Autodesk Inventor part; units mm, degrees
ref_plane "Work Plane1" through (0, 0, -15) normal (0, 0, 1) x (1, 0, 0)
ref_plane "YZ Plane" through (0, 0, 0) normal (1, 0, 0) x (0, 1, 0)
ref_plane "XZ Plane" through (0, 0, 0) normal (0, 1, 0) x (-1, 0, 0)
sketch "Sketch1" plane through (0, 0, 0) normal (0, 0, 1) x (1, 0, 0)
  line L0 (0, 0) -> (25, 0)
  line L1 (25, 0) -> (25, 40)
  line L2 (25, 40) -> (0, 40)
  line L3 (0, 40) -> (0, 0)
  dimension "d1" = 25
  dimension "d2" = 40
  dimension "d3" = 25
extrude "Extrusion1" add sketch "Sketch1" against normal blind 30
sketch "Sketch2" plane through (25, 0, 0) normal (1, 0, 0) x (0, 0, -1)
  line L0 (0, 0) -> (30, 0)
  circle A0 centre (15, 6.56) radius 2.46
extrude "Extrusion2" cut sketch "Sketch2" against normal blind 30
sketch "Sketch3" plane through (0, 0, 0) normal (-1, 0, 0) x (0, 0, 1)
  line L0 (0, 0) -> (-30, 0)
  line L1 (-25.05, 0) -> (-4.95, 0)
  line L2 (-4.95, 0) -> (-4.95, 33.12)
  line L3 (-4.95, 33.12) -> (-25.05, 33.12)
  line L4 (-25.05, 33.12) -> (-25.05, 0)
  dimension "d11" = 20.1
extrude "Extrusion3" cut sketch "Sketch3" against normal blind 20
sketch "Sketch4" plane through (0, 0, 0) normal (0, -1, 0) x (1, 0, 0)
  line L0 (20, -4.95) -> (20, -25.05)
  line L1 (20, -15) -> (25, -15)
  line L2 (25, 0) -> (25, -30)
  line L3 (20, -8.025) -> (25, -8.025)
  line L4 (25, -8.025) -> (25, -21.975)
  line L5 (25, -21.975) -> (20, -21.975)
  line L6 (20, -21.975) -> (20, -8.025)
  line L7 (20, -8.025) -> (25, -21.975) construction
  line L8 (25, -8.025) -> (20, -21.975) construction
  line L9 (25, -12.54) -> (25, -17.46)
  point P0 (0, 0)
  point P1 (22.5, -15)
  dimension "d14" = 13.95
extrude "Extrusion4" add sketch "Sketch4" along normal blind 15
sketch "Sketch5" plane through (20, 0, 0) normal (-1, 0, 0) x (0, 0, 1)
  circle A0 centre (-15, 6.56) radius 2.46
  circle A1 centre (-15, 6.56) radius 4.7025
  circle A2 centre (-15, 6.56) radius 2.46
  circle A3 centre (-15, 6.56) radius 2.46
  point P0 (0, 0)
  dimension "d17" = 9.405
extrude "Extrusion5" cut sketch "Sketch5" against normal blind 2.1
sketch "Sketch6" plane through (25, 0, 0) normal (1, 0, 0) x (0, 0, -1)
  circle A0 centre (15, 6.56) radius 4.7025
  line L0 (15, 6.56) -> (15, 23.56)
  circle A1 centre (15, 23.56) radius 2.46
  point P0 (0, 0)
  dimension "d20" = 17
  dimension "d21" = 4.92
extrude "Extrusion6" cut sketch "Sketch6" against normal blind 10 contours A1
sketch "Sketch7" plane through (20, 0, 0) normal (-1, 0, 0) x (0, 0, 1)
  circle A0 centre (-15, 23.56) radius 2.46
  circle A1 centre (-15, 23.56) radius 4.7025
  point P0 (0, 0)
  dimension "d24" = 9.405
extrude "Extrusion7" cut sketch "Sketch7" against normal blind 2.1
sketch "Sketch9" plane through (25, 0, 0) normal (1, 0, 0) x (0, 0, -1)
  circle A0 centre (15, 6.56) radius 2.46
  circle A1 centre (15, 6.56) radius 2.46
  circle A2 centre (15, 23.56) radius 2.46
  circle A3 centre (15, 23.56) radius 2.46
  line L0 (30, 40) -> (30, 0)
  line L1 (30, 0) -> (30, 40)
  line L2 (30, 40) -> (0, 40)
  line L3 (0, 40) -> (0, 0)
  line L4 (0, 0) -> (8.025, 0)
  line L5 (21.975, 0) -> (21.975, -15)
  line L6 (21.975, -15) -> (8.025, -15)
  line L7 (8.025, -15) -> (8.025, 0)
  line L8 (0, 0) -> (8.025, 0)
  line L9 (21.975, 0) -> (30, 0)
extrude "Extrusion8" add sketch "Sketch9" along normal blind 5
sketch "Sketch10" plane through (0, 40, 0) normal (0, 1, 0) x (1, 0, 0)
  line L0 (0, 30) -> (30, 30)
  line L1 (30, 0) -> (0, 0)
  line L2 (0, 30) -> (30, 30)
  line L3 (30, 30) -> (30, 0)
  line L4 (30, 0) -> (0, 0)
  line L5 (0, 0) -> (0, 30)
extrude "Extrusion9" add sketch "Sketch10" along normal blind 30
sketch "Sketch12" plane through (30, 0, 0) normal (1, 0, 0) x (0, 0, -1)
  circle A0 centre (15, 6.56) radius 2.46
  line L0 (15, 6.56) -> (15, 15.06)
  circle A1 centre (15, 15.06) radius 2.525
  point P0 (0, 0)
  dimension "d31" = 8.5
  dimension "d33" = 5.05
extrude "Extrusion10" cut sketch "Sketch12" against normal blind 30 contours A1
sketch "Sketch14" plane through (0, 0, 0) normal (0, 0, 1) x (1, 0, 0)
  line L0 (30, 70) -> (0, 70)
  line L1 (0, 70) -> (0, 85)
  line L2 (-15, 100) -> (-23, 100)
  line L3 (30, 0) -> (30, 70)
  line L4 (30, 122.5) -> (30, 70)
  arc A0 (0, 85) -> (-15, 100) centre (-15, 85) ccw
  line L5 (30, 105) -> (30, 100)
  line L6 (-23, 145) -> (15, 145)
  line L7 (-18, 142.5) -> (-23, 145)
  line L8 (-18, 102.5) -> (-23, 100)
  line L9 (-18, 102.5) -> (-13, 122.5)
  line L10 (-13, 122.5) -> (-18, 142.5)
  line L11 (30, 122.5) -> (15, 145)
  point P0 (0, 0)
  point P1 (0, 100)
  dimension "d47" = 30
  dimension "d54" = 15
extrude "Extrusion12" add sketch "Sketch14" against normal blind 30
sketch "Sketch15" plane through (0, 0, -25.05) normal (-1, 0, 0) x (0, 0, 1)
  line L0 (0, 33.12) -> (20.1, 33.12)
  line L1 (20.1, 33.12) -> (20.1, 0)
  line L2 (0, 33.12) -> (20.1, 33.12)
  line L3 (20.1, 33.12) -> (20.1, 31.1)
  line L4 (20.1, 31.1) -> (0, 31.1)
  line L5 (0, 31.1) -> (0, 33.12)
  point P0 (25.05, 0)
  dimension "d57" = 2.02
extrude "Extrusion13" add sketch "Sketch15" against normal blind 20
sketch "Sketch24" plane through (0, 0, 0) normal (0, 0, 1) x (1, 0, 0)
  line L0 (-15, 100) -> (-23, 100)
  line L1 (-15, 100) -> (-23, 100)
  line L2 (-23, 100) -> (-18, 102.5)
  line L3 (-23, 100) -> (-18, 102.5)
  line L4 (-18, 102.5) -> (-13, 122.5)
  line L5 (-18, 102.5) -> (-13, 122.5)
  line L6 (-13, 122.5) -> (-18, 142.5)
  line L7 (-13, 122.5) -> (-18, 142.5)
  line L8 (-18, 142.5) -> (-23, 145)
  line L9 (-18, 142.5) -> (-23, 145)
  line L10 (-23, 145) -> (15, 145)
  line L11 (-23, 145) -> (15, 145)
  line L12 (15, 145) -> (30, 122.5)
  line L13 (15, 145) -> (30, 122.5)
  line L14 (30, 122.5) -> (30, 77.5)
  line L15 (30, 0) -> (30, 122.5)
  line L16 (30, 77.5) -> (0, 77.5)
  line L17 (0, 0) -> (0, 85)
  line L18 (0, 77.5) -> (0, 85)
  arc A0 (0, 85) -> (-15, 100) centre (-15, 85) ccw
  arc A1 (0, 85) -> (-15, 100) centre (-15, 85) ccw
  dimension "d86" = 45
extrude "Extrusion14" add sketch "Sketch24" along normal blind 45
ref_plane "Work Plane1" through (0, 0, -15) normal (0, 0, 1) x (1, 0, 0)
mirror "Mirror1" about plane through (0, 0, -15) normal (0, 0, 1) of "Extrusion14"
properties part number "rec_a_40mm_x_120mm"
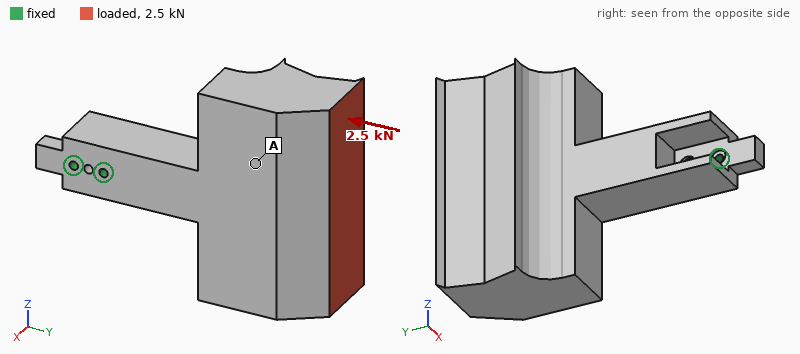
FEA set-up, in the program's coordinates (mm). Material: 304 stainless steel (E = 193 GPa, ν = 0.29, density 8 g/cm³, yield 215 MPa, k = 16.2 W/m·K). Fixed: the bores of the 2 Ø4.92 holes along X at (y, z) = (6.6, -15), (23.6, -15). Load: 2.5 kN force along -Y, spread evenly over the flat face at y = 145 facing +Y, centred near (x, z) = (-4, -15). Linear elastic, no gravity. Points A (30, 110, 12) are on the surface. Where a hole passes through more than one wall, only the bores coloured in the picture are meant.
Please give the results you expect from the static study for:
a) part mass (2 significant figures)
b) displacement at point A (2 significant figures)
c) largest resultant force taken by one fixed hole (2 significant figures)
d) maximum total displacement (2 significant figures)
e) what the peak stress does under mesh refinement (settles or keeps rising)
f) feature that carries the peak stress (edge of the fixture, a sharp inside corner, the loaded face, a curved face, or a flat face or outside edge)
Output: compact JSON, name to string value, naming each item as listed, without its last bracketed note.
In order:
{"part mass": "3.0 kg", "displacement at point A": "61 µm", "largest resultant force taken by one fixed hole": "3.4 kN", "maximum total displacement": "97 µm", "what the peak stress does under mesh refinement": "keeps rising", "feature that carries the peak stress": "edge of the fixture"}
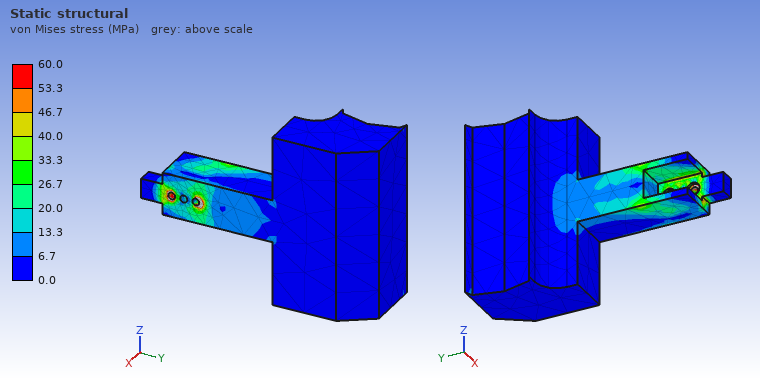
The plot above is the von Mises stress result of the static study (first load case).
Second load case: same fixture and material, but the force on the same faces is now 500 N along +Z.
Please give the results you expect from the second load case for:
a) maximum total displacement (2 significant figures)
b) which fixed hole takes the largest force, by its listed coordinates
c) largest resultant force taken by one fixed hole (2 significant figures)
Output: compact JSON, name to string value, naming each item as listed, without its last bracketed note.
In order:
{"maximum total displacement": "71 µm", "which fixed hole takes the largest force, by its listed coordinates": "(23.6, -15)", "largest resultant force taken by one fixed hole": "3.1 kN"}
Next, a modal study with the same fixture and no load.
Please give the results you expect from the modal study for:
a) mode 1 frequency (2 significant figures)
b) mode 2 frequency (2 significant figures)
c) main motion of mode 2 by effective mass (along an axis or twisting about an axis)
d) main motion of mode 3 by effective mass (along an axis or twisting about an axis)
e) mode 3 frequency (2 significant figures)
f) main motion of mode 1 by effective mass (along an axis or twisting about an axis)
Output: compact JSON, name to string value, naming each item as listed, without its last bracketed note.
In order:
{"mode 1 frequency": "340 Hz", "mode 2 frequency": "370 Hz", "main motion of mode 2 by effective mass": "along Z", "main motion of mode 3 by effective mass": "twisting about Y", "mode 3 frequency": "570 Hz", "main motion of mode 1 by effective mass": "along X"}
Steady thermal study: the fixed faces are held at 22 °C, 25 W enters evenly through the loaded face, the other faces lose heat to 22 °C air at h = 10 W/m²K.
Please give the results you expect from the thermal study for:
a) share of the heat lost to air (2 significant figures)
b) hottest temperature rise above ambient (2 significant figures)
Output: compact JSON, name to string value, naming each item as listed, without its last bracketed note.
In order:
{"share of the heat lost to air": "71 %", "hottest temperature rise above ambient": "74 K"}
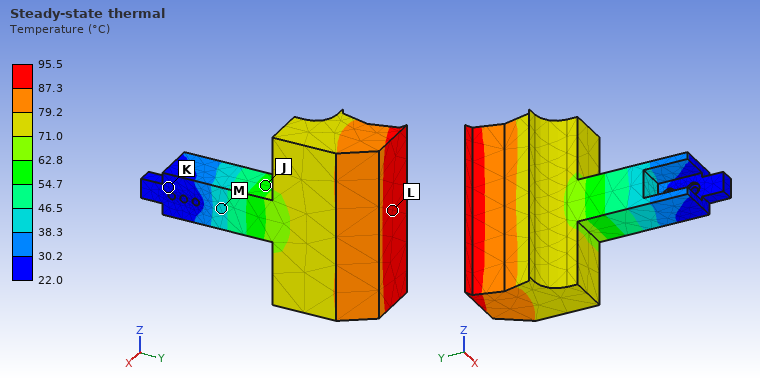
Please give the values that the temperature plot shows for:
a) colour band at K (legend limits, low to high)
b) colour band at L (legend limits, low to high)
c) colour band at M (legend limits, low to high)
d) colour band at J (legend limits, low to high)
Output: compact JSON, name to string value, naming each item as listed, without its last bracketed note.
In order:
{"colour band at K": "22.0 to 30.2 °C", "colour band at L": "87.3 to 95.5 °C", "colour band at M": "38.3 to 46.5 °C", "colour band at J": "54.7 to 62.8 °C"}
